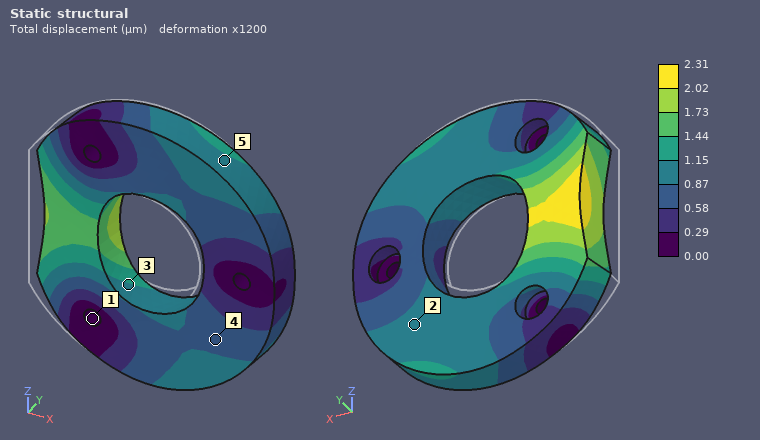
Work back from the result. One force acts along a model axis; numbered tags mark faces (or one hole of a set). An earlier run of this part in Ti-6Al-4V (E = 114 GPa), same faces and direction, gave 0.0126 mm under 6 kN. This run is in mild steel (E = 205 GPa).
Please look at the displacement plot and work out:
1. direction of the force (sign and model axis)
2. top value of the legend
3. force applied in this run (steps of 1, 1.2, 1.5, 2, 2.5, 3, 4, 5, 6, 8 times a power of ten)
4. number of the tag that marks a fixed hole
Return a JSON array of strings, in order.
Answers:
["+X", "2.31 µm", "2 kN", "1"]
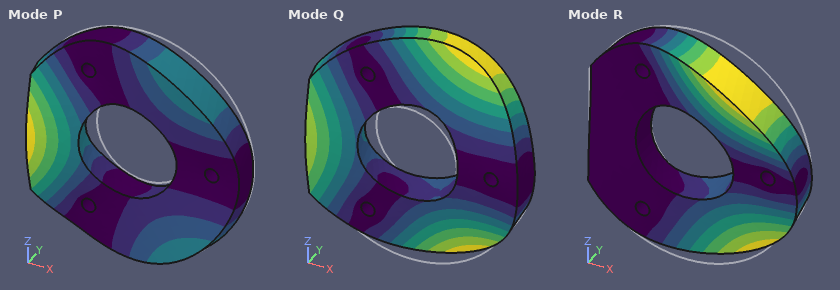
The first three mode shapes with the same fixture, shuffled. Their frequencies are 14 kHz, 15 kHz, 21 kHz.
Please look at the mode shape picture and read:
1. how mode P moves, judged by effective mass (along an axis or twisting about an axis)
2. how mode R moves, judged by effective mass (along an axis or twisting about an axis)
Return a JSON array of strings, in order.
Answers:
["along Y", "twisting about X"]
